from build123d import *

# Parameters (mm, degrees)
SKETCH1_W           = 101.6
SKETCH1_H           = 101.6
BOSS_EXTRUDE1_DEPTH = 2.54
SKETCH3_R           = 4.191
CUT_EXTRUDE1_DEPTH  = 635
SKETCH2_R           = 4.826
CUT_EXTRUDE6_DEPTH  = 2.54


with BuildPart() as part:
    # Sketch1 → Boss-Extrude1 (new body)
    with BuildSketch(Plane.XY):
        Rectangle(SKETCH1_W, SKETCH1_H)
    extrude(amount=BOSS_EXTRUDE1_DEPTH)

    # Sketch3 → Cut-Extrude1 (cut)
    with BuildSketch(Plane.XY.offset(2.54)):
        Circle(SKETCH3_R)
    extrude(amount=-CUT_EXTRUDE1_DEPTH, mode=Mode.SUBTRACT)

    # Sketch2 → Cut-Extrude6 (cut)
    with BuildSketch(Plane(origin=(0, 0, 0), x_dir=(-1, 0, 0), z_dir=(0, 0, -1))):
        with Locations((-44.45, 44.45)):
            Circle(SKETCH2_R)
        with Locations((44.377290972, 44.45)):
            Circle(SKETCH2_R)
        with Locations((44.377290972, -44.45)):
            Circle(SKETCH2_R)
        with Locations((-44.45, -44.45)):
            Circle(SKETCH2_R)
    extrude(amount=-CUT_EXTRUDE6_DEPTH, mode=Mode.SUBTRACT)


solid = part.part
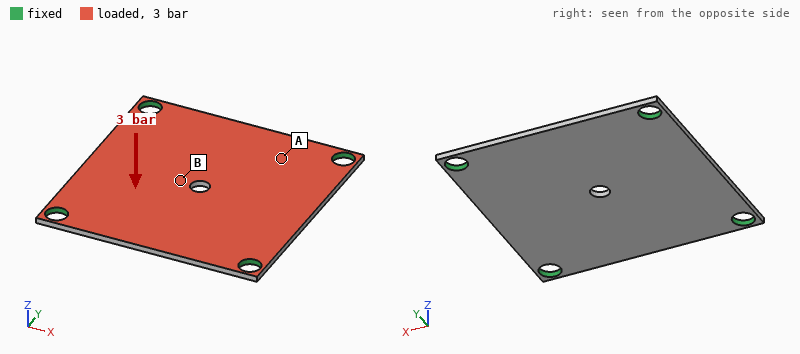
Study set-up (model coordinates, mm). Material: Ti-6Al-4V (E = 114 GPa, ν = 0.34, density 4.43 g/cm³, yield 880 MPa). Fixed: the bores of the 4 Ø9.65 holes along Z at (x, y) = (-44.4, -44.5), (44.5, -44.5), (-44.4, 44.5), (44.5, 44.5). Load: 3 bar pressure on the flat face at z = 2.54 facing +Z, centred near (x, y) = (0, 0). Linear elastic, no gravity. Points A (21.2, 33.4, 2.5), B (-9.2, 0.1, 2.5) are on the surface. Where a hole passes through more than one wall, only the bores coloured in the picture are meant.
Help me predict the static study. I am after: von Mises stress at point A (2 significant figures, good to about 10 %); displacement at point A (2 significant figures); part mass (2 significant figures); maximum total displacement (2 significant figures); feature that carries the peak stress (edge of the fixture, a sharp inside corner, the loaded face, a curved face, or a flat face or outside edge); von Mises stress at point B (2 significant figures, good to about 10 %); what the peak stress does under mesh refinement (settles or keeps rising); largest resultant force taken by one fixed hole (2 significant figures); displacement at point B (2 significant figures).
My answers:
47 MPa
0.28 mm
110 g
0.66 mm
edge of the fixture
110 MPa
keeps rising
750 N
0.63 mm
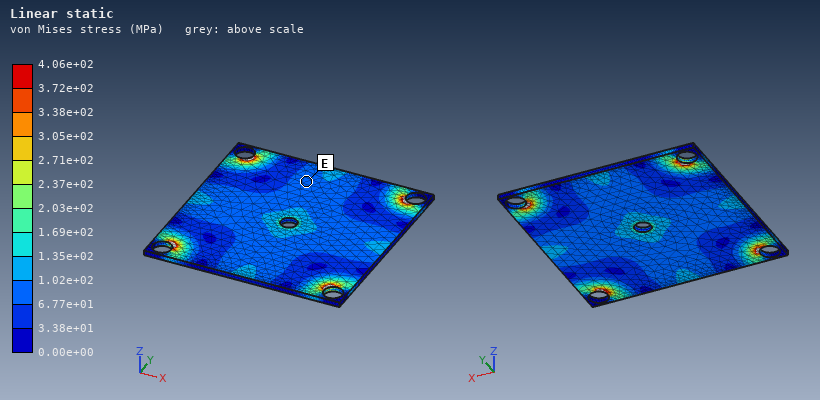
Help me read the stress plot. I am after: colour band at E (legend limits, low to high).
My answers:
6.77e+01 to 1.02e+02 MPa
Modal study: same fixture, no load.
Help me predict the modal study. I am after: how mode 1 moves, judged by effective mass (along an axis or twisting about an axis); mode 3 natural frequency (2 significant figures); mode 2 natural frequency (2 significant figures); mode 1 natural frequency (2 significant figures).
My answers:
along Z
2200 Hz
2200 Hz
1300 Hz
